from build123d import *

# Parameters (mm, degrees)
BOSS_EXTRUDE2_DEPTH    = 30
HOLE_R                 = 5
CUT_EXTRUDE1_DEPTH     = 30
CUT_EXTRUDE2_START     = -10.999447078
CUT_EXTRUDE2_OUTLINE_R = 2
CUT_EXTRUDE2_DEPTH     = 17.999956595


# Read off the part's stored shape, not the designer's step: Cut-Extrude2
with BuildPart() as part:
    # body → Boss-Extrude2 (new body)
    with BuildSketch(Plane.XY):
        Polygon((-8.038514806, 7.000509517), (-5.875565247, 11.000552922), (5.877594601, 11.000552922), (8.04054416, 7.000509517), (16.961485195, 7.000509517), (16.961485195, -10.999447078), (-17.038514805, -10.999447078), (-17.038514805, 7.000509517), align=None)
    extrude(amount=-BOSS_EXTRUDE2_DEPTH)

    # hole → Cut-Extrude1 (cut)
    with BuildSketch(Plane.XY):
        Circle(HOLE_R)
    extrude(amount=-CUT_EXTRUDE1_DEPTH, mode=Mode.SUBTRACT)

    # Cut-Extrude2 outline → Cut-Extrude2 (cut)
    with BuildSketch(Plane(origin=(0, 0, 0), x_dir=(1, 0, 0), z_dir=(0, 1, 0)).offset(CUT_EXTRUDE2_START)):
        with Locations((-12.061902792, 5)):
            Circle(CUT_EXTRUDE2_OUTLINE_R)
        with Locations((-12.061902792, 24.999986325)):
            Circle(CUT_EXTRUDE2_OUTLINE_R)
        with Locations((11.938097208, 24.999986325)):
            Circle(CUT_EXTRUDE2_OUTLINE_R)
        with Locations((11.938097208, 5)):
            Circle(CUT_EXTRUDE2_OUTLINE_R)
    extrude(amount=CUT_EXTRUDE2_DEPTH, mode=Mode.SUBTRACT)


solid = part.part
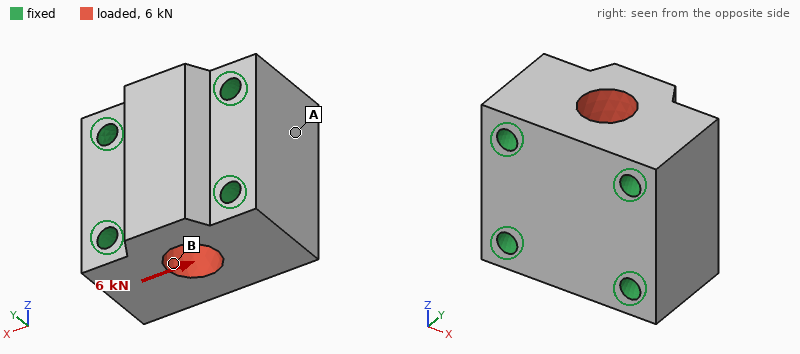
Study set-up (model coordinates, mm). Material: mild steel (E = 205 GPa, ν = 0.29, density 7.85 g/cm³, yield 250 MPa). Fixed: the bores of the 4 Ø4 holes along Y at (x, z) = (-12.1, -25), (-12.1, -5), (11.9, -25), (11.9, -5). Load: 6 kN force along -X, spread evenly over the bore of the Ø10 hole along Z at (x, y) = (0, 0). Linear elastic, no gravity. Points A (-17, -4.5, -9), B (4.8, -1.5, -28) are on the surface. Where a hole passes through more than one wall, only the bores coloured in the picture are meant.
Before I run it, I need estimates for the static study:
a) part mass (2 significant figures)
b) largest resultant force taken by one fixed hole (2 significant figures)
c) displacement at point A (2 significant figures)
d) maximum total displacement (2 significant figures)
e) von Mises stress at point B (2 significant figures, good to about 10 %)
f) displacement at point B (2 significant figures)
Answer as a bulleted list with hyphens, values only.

- 130 g
- 1.5 kN
- 0.14 µm
- 0.57 µm
- 7.5 MPa
- 0.23 µm
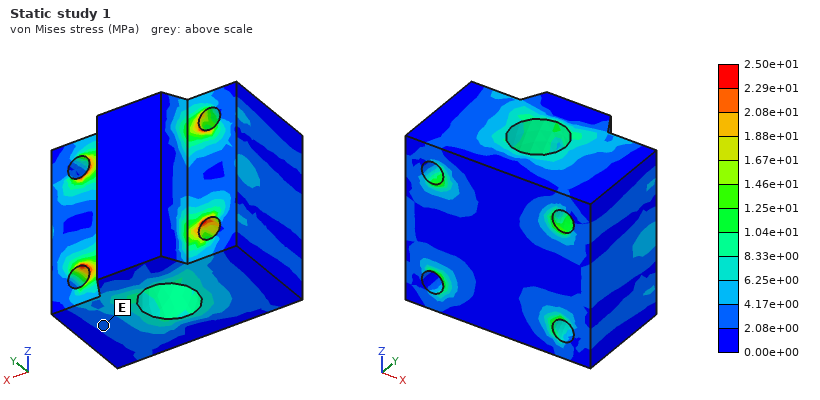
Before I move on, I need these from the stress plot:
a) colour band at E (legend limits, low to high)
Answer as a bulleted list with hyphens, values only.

- 2.08e+00 to 4.17e+00 MPa
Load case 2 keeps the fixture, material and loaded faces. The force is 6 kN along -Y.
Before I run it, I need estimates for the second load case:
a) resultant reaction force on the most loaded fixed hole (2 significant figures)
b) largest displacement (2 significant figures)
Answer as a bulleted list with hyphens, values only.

- 1.5 kN
- 1.0 µm
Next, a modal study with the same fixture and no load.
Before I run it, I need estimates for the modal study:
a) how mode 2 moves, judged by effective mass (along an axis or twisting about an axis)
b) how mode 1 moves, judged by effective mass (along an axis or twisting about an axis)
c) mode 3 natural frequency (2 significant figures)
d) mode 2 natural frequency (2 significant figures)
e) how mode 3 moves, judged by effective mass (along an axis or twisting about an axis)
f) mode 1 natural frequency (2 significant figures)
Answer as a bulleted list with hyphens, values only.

- along Y
- along Z
- 67 kHz
- 57 kHz
- along Z
- 54 kHz
